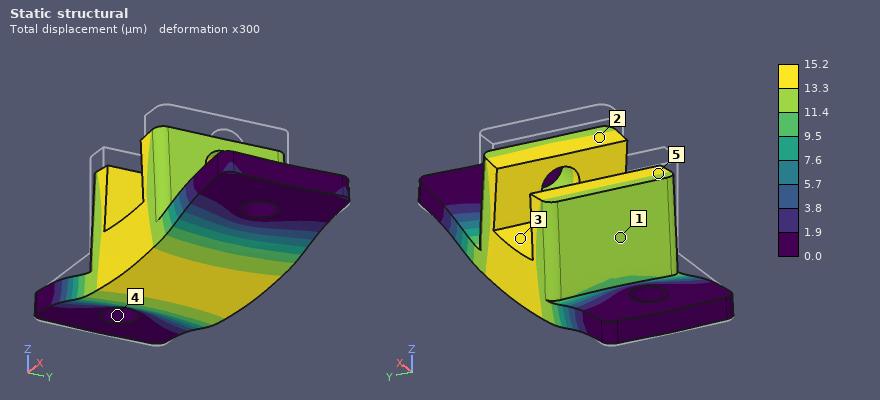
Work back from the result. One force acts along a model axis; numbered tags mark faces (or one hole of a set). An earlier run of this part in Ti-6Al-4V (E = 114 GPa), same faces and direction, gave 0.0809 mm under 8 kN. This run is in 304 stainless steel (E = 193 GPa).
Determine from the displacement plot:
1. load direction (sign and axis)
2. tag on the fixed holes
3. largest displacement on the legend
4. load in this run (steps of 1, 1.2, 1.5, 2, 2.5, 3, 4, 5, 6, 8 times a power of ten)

-Z
4
15.2 µm
2.5 kN
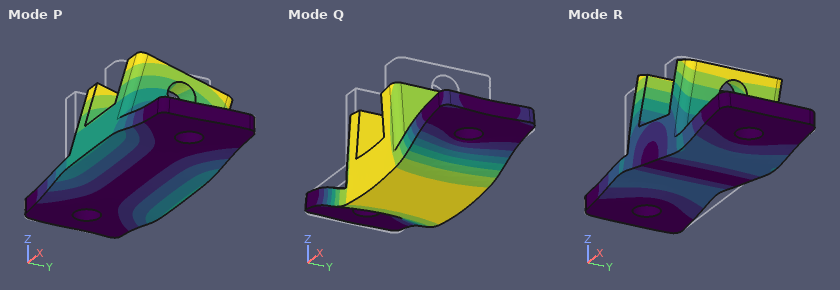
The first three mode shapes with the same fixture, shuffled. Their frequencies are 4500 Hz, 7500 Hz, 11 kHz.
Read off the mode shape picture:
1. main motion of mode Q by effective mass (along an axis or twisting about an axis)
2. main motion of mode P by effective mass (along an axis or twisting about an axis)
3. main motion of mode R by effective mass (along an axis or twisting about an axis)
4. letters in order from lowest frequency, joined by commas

along Z
along Y
along X
P, Q, R
